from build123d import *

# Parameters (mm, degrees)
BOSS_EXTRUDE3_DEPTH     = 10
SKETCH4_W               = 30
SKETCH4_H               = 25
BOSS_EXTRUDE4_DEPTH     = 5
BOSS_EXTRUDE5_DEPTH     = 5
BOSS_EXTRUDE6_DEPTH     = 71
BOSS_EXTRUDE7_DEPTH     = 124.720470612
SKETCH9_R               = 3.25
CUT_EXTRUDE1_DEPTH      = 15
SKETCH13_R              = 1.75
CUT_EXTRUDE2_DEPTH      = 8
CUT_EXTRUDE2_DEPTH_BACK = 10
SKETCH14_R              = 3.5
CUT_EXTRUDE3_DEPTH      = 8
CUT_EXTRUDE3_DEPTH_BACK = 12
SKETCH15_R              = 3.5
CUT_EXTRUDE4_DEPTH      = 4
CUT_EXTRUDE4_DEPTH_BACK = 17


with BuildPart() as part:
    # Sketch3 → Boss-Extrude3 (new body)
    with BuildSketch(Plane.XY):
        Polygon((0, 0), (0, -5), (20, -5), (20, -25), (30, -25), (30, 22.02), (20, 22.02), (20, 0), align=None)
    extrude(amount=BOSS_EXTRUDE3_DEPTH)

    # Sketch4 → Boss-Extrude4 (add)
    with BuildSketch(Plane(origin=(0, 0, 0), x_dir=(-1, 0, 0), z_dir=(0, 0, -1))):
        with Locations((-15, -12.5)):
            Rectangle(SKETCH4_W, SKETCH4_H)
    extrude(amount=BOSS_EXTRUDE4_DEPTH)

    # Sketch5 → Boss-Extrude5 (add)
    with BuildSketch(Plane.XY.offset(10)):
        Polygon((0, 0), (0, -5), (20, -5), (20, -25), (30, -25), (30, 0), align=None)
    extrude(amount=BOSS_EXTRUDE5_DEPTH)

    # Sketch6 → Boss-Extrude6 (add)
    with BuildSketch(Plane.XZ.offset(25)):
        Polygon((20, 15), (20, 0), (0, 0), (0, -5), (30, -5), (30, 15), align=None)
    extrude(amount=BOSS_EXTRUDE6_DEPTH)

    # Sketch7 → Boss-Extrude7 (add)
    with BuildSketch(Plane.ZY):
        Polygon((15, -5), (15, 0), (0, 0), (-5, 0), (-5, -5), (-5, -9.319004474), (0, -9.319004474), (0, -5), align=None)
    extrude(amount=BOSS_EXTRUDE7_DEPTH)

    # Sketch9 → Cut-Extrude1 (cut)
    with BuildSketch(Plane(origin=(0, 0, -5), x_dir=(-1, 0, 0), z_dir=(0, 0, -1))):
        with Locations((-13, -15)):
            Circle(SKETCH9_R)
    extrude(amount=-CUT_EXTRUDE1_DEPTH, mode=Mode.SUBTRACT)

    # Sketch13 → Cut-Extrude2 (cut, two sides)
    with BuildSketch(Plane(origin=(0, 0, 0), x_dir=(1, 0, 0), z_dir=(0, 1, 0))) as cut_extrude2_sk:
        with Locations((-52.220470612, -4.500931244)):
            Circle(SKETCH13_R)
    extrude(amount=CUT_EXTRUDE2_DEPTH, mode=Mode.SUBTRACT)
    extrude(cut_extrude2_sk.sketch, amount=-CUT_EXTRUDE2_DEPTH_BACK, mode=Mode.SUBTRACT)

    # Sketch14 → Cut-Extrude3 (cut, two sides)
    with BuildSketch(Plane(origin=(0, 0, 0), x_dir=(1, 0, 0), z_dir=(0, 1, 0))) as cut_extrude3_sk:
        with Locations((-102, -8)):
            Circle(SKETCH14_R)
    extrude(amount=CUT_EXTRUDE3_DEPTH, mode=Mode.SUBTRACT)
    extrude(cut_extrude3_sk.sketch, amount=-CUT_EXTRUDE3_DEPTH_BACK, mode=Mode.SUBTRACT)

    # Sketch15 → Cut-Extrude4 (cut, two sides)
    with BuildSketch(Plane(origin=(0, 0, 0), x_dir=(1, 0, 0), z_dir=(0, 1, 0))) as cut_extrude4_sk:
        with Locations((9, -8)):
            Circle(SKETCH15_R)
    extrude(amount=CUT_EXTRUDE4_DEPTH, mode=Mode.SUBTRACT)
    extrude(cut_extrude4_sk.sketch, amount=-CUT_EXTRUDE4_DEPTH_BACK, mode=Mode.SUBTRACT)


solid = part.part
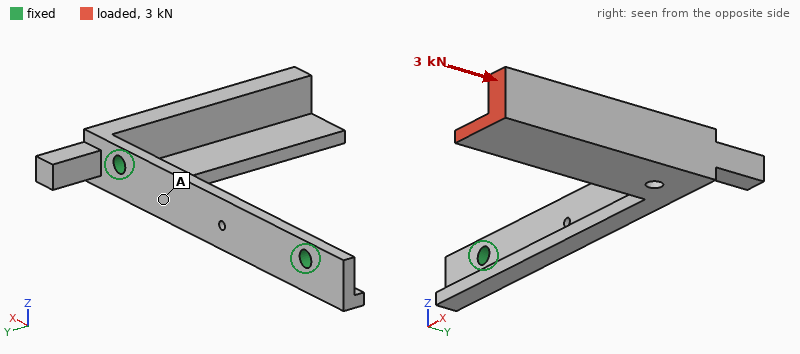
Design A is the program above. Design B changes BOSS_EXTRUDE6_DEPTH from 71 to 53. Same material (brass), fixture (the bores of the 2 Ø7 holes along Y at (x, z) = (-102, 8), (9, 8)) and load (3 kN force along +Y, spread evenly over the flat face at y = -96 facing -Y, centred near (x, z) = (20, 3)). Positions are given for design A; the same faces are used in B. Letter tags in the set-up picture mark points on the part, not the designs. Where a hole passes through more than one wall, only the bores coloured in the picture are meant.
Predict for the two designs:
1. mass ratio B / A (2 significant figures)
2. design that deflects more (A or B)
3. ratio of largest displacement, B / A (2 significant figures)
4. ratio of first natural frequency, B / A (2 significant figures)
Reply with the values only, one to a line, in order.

0.89
A
0.82
1.4
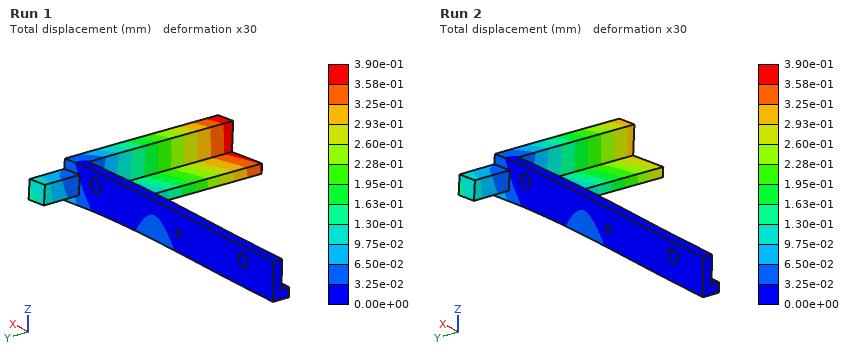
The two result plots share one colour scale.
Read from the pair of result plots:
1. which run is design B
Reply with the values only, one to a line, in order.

Run 2
